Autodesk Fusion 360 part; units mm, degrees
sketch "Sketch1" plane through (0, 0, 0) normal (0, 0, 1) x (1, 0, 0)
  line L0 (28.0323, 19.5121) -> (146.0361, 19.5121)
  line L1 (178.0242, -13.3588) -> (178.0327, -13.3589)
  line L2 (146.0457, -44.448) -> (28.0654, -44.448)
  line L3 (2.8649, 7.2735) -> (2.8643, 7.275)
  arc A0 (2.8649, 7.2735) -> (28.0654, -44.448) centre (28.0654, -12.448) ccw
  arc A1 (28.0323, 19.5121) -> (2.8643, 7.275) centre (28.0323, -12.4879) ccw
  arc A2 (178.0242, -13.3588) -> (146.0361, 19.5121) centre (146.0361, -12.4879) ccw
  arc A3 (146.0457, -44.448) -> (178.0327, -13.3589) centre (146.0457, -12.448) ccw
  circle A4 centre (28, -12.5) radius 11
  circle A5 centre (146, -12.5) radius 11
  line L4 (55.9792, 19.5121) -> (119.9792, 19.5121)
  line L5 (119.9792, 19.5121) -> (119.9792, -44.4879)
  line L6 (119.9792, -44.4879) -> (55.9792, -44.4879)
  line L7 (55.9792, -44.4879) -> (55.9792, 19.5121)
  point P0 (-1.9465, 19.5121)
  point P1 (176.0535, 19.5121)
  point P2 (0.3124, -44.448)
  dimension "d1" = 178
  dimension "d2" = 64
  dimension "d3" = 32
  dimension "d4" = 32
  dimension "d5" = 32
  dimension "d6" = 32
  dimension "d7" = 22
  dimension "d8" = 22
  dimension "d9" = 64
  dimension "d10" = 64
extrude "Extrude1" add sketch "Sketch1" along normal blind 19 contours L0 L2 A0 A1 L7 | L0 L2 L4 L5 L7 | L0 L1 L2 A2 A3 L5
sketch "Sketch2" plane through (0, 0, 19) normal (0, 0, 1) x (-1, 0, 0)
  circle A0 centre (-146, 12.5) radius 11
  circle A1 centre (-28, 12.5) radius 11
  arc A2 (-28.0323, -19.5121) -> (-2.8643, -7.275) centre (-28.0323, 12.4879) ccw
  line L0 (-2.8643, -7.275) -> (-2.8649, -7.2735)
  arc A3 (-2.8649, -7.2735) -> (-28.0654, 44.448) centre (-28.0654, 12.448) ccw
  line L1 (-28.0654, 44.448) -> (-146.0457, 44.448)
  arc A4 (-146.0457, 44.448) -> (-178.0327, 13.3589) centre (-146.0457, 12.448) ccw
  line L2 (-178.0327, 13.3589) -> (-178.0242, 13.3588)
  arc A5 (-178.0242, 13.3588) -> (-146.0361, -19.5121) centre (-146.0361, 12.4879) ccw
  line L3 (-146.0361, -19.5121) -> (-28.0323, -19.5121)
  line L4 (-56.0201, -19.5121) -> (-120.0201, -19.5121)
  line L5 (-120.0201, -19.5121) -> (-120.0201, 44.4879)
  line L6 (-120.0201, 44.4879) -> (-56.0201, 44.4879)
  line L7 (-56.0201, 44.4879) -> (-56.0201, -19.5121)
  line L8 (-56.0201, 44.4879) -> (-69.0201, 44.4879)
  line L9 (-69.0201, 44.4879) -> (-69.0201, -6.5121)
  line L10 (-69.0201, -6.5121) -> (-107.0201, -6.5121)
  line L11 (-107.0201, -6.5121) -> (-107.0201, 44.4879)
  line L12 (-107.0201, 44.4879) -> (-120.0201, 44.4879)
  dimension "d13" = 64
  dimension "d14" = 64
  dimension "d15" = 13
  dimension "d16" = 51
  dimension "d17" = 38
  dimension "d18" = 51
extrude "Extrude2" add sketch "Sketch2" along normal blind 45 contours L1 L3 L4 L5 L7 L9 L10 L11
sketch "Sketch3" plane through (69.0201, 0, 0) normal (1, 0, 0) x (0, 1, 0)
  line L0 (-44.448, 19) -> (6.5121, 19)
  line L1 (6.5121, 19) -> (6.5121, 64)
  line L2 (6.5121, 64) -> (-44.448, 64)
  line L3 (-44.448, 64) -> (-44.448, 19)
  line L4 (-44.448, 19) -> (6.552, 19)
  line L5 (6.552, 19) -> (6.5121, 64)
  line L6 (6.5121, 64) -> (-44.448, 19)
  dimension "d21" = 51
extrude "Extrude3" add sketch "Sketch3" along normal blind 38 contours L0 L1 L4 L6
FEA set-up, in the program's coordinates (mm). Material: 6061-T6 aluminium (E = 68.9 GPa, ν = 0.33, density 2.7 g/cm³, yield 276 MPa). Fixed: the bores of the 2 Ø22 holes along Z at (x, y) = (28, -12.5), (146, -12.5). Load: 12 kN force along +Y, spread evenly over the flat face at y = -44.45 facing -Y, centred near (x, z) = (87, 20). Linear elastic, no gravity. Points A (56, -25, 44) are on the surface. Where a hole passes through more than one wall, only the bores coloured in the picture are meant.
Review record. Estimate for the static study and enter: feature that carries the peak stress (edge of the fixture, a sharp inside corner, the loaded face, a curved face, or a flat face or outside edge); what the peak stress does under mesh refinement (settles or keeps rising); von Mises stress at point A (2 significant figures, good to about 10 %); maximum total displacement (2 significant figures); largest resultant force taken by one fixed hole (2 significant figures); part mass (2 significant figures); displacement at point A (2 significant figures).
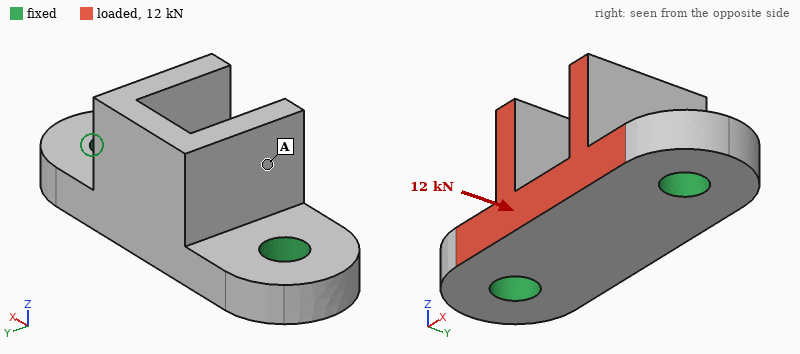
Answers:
edge of the fixture
keeps rising
4.1 MPa
38 µm
6.1 kN
890 g
25 µm
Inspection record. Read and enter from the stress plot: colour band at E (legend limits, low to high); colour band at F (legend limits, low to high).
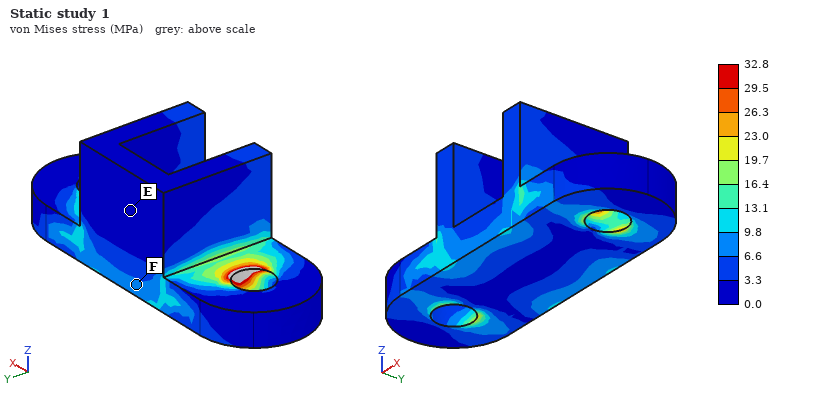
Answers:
0.0 to 3.3 MPa
6.6 to 9.8 MPa
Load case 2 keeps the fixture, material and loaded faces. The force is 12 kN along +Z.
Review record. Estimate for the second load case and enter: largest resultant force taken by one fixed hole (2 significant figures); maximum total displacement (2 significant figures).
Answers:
6.3 kN
77 µm
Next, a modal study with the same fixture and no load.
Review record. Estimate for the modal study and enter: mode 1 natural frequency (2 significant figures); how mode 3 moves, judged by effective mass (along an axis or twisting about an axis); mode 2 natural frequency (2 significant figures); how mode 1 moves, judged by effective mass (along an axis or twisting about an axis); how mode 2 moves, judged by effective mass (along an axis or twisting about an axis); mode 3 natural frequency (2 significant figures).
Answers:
3400 Hz
along X
5900 Hz
along Y
along Z
6900 Hz
